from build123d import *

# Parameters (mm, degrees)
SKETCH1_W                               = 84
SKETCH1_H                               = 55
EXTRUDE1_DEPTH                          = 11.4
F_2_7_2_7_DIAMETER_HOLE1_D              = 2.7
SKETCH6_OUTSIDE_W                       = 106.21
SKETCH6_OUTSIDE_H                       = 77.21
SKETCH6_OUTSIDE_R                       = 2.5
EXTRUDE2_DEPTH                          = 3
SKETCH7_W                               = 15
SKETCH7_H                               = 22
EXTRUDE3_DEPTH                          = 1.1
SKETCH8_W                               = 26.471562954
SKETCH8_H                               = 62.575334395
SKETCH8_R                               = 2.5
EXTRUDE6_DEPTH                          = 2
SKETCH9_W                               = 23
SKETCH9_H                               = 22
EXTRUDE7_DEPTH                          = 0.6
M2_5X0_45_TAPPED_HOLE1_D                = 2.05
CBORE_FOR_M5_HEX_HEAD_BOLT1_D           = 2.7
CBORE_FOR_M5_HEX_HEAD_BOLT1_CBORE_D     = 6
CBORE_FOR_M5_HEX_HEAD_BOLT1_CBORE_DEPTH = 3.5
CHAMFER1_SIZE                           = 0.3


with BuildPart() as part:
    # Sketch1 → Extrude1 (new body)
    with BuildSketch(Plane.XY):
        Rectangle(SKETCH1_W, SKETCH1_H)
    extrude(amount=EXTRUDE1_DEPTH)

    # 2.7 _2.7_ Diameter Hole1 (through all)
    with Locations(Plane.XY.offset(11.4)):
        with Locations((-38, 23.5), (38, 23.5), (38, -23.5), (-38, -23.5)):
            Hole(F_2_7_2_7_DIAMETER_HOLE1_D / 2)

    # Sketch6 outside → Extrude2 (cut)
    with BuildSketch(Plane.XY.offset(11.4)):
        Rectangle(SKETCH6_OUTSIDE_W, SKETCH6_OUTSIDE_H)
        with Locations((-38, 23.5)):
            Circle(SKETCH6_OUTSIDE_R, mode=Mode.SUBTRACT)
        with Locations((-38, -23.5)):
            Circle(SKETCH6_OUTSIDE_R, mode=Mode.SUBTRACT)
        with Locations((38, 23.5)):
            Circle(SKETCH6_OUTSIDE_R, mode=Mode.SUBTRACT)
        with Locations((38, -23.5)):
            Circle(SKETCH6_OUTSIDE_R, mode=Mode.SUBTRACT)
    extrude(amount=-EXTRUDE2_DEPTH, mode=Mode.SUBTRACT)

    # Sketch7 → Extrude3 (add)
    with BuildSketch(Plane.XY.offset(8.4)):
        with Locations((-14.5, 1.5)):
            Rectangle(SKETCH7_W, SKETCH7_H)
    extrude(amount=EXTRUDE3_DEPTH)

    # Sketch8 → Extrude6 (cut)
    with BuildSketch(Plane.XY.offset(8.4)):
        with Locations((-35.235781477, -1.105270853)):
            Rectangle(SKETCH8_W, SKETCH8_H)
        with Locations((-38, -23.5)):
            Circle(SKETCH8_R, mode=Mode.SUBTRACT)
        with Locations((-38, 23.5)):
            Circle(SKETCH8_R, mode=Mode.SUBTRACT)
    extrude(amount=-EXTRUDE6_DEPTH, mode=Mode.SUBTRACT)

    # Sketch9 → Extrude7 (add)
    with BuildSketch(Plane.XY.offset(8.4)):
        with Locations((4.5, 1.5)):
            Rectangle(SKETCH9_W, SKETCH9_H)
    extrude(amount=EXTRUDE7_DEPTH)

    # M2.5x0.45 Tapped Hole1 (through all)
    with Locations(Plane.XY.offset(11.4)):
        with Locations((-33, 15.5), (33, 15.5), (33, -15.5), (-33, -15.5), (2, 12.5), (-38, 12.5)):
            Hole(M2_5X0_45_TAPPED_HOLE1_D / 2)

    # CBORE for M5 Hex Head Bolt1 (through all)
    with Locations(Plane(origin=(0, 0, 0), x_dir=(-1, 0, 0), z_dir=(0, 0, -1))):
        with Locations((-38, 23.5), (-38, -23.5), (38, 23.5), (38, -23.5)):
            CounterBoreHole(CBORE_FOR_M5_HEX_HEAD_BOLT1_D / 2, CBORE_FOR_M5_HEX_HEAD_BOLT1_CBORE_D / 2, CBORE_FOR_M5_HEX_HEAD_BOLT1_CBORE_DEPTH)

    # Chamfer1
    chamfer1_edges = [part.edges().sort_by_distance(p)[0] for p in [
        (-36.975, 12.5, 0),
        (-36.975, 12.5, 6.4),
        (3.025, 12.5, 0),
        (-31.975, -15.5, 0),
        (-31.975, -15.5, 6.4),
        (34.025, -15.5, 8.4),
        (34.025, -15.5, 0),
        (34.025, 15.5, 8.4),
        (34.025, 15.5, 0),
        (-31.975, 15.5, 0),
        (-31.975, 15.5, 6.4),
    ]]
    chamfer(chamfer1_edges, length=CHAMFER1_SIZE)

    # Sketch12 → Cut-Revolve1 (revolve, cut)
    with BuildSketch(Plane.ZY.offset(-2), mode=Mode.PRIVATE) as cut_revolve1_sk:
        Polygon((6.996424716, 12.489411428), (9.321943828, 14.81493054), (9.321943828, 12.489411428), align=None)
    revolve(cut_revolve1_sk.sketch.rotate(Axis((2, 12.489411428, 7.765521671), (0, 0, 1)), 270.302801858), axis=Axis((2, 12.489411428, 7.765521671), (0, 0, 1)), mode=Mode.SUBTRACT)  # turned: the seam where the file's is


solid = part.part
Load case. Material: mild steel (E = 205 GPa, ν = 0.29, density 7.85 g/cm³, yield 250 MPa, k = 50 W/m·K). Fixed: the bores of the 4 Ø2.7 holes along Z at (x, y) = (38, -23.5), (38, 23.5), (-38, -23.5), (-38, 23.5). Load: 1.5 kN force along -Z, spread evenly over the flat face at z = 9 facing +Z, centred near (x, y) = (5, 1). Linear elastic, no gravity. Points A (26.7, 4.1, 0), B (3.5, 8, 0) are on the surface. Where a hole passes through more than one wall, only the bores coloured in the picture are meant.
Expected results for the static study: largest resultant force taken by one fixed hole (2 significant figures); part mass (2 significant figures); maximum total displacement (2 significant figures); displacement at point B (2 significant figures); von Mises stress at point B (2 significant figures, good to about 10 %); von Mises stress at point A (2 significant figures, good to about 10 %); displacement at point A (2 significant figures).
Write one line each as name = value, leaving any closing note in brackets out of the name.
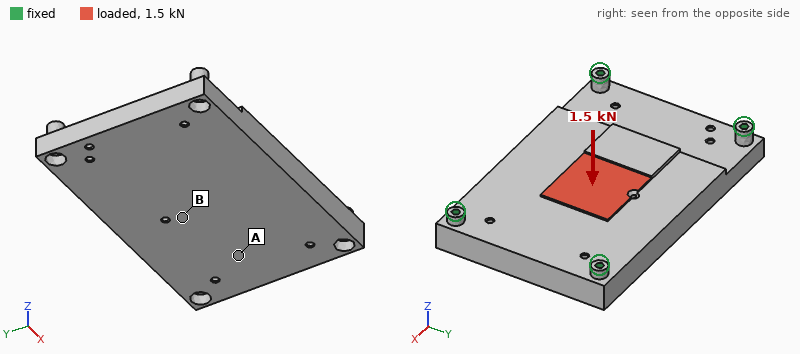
largest resultant force taken by one fixed hole = 600 N
part mass = 290 g
maximum total displacement = 15 µm
displacement at point B = 15 µm
von Mises stress at point B = 26 MPa
von Mises stress at point A = 9.6 MPa
displacement at point A = 7.4 µm
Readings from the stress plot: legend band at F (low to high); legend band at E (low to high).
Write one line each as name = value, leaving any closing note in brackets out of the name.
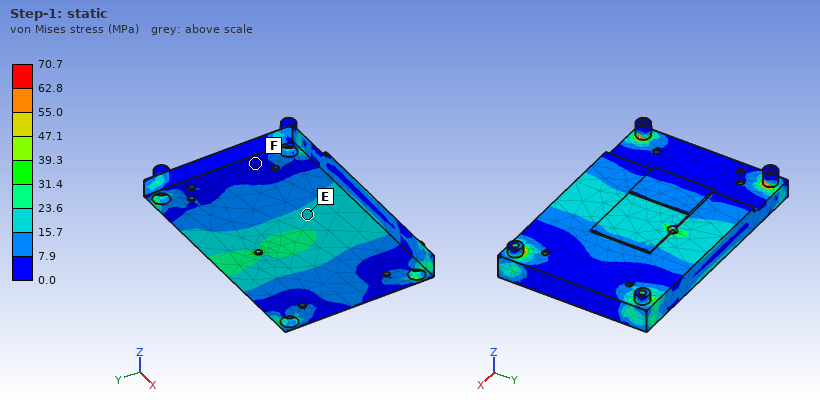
legend band at F = 0.0 to 7.9 MPa
legend band at E = 15.7 to 23.6 MPa
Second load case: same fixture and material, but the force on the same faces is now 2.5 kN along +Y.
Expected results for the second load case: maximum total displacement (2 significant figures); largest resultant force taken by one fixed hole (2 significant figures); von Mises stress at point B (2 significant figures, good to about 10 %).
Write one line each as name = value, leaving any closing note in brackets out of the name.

maximum total displacement = 5.8 µm
largest resultant force taken by one fixed hole = 880 N
von Mises stress at point B = 4.2 MPa
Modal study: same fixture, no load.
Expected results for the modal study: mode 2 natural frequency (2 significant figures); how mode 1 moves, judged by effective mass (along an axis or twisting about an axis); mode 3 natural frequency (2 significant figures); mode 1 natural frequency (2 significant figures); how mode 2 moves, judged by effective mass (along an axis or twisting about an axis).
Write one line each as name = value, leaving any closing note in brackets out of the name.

mode 2 natural frequency = 7200 Hz
how mode 1 moves, judged by effective mass = along Z
mode 3 natural frequency = 10 kHz
mode 1 natural frequency = 4200 Hz
how mode 2 moves, judged by effective mass = twisting about X
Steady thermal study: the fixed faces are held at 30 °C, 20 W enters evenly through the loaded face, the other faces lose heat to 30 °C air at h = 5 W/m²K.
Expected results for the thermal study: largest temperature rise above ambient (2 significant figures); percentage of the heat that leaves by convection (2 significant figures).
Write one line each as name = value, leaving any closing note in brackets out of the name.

largest temperature rise above ambient = 28 K
percentage of the heat that leaves by convection = 4.2 %
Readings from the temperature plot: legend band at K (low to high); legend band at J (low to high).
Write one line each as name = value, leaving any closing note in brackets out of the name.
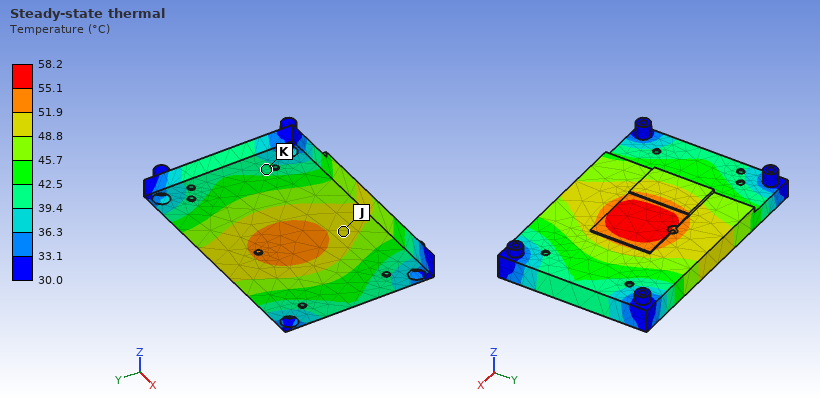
legend band at K = 39.4 to 42.5 °C
legend band at J = 48.8 to 51.9 °C
